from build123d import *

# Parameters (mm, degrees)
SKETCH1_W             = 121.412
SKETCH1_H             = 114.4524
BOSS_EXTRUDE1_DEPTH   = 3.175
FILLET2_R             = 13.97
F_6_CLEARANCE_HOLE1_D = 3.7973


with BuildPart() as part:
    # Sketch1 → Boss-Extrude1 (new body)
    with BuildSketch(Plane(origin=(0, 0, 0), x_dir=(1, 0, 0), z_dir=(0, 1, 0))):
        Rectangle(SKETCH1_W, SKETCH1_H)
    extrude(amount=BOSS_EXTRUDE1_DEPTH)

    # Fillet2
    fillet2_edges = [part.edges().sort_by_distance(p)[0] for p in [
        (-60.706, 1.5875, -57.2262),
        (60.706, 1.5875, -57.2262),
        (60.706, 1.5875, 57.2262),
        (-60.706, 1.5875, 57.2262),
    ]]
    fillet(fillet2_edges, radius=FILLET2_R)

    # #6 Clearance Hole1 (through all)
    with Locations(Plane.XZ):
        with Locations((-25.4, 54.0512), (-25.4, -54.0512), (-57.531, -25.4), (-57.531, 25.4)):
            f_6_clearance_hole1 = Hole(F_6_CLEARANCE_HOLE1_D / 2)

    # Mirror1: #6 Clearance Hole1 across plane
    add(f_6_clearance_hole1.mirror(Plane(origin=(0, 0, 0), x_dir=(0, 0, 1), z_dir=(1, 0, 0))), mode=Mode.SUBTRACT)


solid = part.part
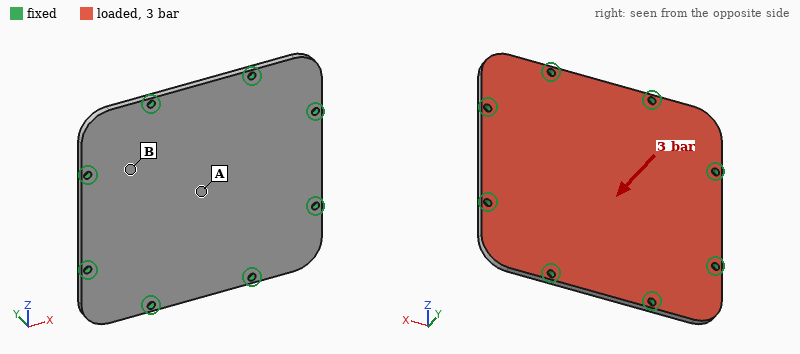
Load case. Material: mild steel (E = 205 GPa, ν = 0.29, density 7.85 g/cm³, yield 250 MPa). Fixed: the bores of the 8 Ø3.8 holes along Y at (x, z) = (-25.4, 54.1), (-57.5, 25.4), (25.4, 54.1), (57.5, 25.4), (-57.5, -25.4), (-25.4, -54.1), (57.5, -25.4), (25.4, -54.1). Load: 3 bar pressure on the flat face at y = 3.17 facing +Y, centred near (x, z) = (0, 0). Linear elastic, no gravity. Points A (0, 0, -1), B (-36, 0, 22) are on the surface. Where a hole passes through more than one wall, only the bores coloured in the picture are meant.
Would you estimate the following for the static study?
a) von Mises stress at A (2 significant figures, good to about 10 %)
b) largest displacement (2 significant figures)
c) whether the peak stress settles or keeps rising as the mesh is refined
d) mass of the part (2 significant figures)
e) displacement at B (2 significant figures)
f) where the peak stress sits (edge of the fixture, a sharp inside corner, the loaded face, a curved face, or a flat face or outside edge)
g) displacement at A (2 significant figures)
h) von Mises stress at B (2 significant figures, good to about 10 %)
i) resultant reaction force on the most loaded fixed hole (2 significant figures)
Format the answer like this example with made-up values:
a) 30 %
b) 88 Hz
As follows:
a) 64 MPa
b) 0.15 mm
c) keeps rising
d) 340 g
e) 0.056 mm
f) edge of the fixture
g) 0.15 mm
h) 28 MPa
i) 530 N
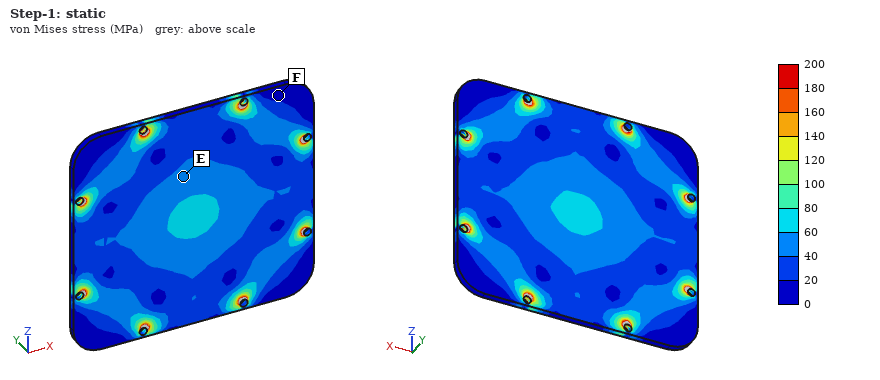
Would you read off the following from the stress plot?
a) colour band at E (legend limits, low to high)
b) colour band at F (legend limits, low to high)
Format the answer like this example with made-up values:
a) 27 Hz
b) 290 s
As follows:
a) 40 to 60 MPa
b) 0 to 20 MPa
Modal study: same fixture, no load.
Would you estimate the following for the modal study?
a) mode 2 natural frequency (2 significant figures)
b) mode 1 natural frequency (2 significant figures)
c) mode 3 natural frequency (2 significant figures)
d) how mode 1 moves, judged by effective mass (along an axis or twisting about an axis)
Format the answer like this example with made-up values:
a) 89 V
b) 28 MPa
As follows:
a) 3600 Hz
b) 1700 Hz
c) 3800 Hz
d) along Y
